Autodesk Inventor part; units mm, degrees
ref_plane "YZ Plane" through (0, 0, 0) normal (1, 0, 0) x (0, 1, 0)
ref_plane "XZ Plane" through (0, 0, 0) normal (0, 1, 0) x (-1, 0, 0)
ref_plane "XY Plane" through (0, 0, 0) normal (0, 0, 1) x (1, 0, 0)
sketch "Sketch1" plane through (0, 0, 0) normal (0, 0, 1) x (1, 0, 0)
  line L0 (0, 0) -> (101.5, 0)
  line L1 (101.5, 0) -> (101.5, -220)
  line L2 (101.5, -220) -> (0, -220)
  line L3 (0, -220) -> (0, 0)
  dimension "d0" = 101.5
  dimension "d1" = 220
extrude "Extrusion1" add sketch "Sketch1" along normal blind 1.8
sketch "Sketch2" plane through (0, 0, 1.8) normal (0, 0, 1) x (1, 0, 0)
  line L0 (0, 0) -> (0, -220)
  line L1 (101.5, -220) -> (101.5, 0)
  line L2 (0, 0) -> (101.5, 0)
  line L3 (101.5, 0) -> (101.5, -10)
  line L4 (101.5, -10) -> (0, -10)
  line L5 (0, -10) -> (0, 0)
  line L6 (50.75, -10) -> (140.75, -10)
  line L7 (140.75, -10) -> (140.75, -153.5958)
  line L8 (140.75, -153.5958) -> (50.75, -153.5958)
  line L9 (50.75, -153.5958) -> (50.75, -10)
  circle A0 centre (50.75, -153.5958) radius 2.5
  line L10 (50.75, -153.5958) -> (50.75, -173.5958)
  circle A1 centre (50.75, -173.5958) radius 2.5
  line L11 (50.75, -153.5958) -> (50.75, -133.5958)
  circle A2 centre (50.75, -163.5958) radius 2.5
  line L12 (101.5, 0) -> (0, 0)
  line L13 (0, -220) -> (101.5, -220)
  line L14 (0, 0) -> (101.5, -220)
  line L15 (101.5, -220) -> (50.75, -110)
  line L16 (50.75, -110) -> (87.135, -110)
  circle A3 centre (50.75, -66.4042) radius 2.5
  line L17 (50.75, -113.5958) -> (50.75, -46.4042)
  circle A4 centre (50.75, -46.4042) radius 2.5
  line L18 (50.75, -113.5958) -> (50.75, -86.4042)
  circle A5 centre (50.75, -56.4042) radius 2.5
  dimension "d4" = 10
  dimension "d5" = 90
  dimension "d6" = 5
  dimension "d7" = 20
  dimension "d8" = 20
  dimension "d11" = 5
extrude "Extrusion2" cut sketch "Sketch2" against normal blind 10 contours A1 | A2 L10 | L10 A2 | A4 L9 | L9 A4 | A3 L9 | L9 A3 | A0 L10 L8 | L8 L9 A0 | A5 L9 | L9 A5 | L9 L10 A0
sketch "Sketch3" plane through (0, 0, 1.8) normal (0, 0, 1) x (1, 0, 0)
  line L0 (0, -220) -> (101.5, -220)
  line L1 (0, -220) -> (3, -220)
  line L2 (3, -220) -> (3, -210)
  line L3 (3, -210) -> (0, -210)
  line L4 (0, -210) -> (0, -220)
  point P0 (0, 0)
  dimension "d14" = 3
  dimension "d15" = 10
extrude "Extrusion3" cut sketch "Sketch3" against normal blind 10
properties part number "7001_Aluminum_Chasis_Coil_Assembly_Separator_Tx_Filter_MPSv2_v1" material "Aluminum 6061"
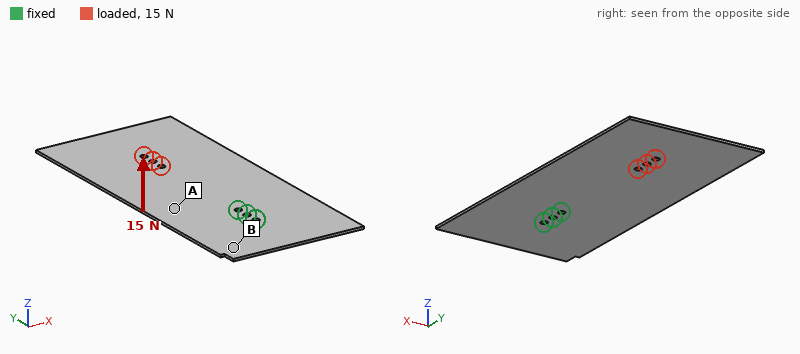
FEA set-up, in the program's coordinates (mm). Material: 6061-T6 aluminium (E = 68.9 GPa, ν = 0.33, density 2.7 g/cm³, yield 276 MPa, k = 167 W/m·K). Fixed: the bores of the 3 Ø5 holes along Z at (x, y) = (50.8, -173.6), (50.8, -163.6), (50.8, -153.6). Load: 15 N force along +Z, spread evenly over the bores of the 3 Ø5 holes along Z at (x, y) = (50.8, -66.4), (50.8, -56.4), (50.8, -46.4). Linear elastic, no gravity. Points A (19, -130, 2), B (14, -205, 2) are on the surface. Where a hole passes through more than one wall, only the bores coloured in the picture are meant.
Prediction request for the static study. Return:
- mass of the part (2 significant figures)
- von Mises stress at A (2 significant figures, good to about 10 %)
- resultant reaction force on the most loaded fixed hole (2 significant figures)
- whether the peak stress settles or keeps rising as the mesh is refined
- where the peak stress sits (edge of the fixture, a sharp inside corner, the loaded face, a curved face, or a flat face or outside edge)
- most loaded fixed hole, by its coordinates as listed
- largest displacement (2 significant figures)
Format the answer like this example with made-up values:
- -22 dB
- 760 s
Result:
- 110 g
- 19 MPa
- 64 N
- keeps rising
- edge of the fixture
- (50.8, -153.6)
- 2.8 mm
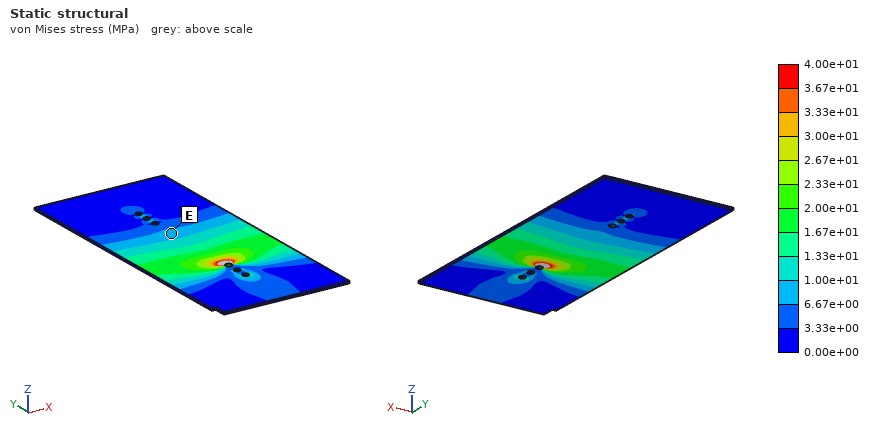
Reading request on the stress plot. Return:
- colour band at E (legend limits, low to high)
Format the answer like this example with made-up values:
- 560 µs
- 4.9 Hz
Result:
- 6.67e+00 to 1.00e+01 MPa
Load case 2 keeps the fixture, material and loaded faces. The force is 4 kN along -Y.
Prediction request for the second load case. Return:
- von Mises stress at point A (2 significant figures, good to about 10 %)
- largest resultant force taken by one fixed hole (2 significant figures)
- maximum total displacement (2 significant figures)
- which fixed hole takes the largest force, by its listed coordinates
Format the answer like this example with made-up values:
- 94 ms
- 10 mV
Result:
- 18 MPa
- 2.0 kN
- 63 µm
- (50.8, -153.6)
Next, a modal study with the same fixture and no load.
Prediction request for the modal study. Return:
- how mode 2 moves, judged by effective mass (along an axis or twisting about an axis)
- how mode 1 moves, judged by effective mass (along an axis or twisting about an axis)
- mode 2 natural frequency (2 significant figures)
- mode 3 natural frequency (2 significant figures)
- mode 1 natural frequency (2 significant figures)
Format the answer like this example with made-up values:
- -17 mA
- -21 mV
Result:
- twisting about Y
- along Z
- 170 Hz
- 350 Hz
- 60 Hz
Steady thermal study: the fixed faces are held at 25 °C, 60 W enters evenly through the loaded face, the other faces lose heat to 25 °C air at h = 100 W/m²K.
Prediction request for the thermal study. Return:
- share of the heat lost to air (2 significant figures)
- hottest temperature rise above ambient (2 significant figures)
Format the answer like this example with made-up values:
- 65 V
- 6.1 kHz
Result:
- 96 %
- 72 K
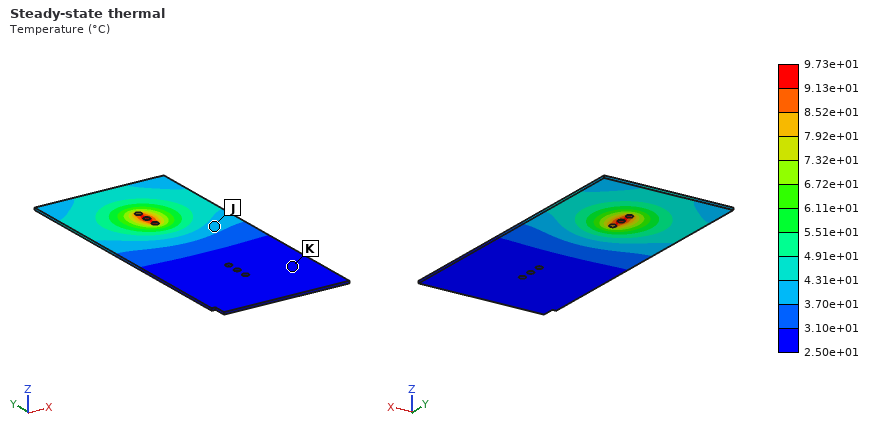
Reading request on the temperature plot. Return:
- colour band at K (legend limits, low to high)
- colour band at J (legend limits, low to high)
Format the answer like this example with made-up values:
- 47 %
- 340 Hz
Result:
- 2.50e+01 to 3.10e+01 °C
- 3.70e+01 to 4.31e+01 °C
